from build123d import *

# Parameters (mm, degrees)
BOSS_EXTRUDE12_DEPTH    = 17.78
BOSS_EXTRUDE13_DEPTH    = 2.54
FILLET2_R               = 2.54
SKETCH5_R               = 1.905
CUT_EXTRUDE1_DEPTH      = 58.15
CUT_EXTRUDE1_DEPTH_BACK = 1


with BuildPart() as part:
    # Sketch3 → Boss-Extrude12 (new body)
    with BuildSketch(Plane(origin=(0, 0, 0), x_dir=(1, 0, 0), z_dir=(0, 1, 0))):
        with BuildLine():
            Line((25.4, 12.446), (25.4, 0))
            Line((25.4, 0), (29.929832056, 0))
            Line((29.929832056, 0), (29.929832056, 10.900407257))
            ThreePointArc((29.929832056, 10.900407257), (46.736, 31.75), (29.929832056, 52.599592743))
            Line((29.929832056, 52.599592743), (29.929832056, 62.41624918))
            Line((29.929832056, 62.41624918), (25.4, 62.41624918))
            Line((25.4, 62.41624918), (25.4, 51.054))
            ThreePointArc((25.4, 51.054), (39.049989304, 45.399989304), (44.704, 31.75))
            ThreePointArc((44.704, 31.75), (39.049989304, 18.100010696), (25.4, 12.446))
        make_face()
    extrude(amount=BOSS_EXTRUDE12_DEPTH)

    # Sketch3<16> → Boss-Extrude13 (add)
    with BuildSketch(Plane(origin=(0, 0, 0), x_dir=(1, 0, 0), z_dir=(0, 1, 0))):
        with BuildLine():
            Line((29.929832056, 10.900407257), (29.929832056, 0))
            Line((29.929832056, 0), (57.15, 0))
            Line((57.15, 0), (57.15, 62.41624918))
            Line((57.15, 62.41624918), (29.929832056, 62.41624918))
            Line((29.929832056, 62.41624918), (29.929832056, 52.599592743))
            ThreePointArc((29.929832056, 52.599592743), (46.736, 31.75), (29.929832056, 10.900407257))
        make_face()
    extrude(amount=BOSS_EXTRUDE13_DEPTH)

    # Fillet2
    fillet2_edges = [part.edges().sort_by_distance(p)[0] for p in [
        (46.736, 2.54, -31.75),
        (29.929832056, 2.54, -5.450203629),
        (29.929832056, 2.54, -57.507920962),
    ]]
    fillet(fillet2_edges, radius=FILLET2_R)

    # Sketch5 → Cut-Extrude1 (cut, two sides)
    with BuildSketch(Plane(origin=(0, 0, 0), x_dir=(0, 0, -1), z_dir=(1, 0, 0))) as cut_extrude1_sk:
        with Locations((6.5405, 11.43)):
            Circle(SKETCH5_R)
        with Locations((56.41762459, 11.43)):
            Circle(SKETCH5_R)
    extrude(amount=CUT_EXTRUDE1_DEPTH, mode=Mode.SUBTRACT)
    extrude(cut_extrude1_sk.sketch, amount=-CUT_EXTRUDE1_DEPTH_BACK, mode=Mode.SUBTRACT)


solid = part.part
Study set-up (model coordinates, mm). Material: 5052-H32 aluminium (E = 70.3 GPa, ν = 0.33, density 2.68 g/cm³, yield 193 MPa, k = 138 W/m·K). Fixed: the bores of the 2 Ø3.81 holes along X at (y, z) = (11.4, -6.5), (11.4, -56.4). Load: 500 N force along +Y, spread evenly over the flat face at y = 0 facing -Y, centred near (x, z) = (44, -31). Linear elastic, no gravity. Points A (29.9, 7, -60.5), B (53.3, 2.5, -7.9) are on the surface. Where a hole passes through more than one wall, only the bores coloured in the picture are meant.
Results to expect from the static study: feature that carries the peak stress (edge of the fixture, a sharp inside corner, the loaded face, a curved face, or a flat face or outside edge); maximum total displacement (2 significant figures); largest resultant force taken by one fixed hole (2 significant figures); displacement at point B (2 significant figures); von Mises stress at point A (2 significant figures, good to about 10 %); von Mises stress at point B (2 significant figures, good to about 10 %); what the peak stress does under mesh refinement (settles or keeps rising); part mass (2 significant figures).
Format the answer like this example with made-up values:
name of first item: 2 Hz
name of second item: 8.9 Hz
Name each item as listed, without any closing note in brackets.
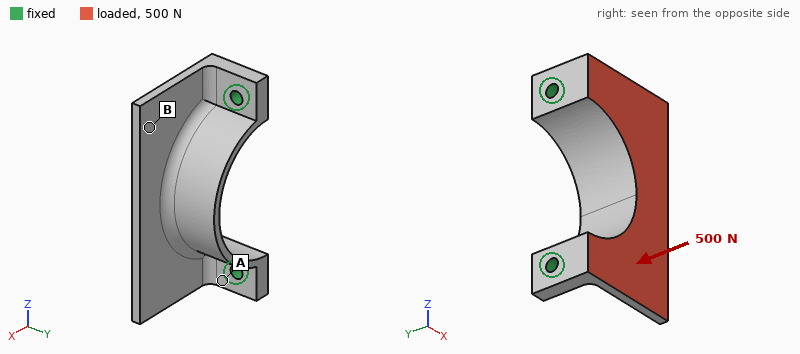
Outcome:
feature that carries the peak stress: edge of the fixture
maximum total displacement: 0.14 mm
largest resultant force taken by one fixed hole: 260 N
displacement at point B: 0.10 mm
von Mises stress at point A: 33 MPa
von Mises stress at point B: 7.5 MPa
what the peak stress does under mesh refinement: keeps rising
part mass: 19 g
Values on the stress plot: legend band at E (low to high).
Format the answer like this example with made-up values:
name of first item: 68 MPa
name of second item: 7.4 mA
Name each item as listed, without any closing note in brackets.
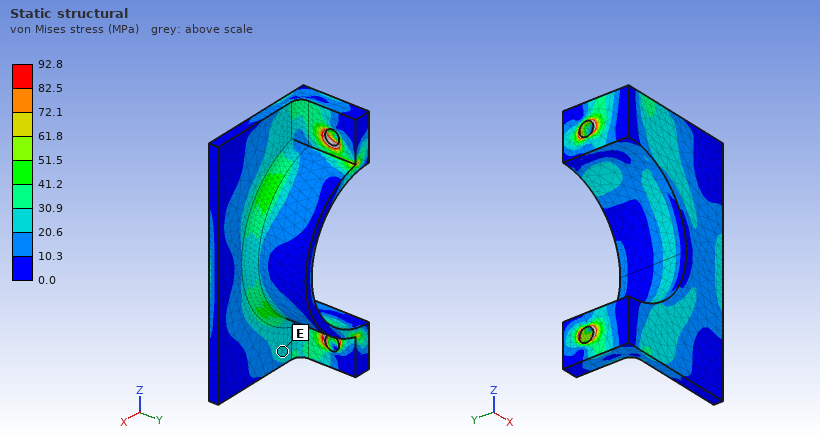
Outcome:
legend band at E: 20.6 to 30.9 MPa
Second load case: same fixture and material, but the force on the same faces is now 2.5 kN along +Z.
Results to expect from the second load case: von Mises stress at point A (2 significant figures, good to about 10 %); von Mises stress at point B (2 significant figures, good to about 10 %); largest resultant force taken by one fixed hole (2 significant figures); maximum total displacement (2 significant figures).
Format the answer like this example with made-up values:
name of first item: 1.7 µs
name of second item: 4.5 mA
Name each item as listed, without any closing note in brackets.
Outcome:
von Mises stress at point A: 53 MPa
von Mises stress at point B: 18 MPa
largest resultant force taken by one fixed hole: 1.5 kN
maximum total displacement: 73 µm
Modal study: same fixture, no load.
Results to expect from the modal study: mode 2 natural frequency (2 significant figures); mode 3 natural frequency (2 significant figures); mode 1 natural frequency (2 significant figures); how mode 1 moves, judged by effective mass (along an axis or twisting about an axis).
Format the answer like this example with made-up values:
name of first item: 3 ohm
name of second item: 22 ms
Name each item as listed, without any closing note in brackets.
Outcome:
mode 2 natural frequency: 4500 Hz
mode 3 natural frequency: 7700 Hz
mode 1 natural frequency: 3900 Hz
how mode 1 moves, judged by effective mass: along Y
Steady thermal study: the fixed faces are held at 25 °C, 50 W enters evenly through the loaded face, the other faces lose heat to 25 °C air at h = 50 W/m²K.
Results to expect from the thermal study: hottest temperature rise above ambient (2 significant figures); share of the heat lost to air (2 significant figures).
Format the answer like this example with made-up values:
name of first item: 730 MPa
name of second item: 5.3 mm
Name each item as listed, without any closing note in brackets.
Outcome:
hottest temperature rise above ambient: 53 K
share of the heat lost to air: 13 %
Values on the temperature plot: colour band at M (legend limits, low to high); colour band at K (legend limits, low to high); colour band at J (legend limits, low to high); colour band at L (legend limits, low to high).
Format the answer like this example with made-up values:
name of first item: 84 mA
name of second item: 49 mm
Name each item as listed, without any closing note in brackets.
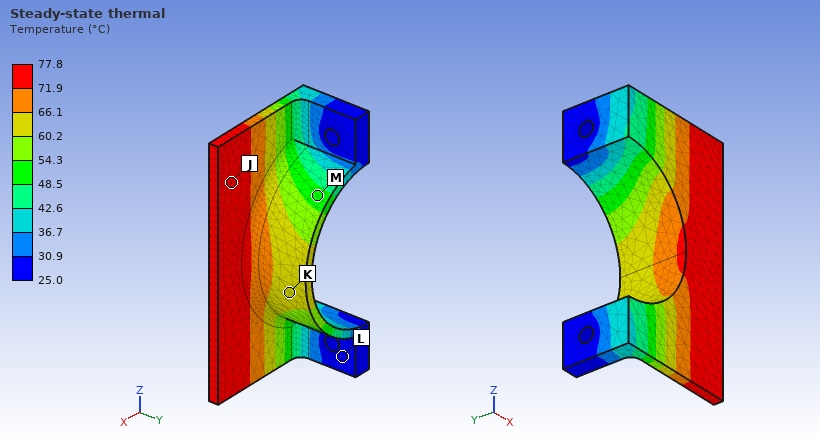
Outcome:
colour band at M: 48.5 to 54.3 °C
colour band at K: 60.2 to 66.1 °C
colour band at J: 71.9 to 77.8 °C
colour band at L: 25.0 to 30.9 °C
